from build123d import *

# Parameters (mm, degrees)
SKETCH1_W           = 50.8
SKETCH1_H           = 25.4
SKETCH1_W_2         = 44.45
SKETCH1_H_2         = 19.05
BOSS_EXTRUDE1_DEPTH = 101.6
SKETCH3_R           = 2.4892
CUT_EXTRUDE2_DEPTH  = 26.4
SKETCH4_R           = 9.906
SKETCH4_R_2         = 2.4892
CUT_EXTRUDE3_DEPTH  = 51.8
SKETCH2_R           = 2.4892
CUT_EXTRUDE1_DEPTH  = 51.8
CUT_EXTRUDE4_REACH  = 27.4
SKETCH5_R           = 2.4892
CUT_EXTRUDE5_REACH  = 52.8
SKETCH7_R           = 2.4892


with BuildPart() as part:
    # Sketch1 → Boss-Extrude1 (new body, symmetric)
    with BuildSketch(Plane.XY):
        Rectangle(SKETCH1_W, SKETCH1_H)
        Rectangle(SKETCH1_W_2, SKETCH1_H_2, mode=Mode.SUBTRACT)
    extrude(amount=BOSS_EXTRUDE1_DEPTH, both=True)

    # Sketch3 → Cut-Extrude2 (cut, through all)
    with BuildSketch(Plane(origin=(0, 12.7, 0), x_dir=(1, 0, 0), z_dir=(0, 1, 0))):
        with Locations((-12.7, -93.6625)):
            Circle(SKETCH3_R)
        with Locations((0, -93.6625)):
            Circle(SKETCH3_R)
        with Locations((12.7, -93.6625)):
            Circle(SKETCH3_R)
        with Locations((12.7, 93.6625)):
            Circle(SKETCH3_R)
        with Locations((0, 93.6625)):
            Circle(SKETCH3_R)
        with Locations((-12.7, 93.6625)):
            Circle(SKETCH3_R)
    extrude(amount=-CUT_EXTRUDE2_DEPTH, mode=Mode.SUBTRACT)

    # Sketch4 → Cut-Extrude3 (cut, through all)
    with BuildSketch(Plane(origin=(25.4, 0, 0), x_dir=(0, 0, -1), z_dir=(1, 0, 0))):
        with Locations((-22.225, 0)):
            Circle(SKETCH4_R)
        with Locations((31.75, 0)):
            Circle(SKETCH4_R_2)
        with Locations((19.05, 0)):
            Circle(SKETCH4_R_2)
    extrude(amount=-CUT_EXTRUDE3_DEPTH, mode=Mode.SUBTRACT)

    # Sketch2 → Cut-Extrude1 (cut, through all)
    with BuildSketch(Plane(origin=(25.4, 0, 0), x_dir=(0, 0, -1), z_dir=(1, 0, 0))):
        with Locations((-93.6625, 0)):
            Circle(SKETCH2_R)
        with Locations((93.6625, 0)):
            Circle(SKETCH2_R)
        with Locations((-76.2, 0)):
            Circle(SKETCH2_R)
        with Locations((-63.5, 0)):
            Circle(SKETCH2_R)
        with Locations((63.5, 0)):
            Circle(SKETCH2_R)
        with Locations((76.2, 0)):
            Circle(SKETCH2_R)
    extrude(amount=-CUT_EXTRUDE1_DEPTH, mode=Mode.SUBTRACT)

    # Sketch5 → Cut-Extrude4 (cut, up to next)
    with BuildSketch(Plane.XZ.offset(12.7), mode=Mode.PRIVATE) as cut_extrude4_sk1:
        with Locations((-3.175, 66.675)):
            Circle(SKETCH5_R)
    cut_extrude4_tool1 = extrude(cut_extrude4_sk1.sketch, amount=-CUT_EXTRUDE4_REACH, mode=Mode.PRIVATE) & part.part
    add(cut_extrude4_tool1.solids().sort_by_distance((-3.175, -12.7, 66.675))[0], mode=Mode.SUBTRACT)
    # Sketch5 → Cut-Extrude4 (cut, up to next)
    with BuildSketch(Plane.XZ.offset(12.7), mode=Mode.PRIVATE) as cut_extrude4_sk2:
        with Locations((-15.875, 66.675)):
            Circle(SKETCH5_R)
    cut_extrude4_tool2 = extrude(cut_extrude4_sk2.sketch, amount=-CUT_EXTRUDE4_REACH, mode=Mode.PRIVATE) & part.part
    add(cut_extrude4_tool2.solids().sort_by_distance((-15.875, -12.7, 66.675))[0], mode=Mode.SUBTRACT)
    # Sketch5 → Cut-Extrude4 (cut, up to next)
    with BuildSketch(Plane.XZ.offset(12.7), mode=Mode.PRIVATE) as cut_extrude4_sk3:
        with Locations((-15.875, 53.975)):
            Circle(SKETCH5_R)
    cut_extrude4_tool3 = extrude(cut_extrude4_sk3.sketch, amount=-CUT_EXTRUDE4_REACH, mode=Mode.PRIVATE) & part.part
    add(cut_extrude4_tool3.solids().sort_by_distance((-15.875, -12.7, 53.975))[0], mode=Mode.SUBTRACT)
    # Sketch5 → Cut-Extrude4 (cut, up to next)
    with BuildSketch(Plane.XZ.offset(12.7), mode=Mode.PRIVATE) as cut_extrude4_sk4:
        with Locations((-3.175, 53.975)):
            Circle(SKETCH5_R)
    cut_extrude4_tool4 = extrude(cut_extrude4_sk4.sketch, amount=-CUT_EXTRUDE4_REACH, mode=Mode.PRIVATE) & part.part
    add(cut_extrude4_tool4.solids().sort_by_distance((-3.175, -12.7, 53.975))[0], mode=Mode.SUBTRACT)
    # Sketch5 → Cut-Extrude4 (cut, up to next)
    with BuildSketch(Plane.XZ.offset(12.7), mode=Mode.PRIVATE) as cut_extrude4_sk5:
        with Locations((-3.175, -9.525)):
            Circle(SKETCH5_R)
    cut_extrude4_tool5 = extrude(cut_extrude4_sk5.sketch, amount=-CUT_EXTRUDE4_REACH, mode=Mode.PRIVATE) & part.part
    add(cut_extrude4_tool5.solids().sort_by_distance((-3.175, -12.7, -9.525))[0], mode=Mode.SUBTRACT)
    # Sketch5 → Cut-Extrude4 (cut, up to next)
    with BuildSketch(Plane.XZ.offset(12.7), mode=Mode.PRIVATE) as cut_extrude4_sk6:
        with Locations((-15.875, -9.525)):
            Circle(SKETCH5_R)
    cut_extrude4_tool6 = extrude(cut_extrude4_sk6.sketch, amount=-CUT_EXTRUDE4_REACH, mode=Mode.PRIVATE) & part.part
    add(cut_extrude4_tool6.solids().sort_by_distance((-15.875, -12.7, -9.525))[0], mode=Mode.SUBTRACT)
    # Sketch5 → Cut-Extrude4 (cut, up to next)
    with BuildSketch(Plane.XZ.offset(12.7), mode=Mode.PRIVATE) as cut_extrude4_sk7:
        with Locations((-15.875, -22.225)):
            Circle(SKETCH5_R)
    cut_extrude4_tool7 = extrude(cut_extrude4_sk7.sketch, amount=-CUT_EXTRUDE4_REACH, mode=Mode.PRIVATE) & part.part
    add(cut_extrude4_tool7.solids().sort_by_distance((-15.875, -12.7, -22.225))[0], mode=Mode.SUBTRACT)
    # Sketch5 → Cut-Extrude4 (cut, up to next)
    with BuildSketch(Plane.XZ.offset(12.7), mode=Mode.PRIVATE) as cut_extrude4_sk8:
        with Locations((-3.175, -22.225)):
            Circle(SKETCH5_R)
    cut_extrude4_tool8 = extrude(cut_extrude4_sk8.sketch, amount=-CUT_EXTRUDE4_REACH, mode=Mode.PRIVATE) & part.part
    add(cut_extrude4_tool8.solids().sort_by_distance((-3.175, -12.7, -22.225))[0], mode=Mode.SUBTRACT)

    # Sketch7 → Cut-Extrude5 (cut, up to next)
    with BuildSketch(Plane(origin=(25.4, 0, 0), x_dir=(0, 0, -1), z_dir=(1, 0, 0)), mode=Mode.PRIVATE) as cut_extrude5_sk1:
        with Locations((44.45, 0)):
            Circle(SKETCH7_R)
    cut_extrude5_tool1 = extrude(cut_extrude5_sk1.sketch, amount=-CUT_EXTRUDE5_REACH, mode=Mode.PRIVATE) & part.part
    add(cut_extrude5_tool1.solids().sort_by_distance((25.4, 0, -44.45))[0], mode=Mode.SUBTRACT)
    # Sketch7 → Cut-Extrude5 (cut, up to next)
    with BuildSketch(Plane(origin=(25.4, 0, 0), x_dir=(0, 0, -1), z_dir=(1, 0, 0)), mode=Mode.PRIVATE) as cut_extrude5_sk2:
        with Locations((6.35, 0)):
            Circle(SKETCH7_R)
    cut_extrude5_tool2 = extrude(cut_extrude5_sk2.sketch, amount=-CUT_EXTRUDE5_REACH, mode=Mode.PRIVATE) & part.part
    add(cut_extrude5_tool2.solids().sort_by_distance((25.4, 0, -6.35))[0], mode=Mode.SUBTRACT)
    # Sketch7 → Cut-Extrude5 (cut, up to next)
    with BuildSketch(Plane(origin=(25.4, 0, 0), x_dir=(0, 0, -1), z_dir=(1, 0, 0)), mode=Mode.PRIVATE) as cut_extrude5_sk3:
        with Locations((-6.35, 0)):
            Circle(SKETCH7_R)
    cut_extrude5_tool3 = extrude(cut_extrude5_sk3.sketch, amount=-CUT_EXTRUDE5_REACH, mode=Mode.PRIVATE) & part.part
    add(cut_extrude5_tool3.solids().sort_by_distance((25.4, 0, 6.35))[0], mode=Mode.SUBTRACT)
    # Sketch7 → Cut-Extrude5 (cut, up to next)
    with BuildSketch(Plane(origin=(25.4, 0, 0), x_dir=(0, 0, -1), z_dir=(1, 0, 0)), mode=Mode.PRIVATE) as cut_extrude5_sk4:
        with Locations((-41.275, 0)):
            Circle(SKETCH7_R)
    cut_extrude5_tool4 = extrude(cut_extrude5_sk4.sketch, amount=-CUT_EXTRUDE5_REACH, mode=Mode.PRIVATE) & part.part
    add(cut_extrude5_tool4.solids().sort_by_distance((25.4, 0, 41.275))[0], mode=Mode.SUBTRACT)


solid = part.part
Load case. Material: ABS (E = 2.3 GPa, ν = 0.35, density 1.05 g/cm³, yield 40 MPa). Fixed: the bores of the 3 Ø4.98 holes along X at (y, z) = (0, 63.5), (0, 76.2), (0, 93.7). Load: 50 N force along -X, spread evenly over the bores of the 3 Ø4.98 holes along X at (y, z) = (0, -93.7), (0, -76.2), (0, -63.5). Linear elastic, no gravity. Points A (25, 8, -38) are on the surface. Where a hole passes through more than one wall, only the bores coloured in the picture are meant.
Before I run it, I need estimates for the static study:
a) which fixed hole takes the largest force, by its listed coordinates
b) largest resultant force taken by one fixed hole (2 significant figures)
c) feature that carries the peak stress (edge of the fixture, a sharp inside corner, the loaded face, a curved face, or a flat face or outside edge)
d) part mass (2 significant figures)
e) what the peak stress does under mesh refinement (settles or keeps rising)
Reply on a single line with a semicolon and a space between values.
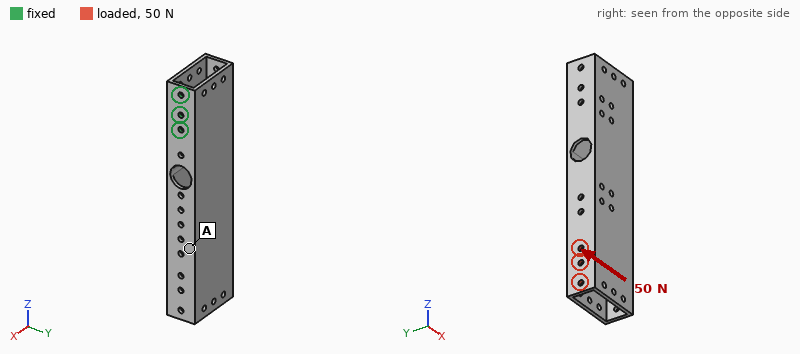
(0, 63.5); 250 N; edge of the fixture; 90 g; keeps rising
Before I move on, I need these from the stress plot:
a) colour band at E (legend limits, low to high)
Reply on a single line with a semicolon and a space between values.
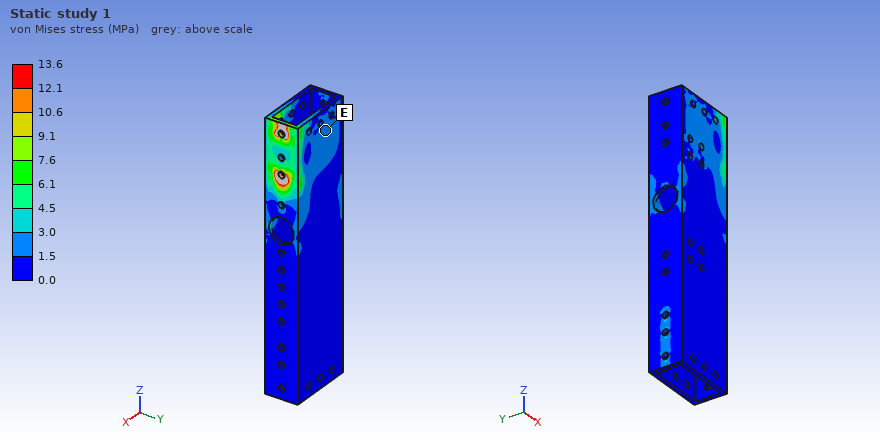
1.5 to 3.0 MPa
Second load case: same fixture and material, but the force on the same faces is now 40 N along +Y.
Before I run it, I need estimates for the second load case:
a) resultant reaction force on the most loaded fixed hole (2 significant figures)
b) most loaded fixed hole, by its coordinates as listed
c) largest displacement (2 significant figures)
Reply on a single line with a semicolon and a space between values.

210 N; (0, 63.5); 2.3 mm
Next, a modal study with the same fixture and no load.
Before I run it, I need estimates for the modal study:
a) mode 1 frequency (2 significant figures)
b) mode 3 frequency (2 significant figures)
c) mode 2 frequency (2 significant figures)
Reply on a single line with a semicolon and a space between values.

130 Hz; 230 Hz; 130 Hz
